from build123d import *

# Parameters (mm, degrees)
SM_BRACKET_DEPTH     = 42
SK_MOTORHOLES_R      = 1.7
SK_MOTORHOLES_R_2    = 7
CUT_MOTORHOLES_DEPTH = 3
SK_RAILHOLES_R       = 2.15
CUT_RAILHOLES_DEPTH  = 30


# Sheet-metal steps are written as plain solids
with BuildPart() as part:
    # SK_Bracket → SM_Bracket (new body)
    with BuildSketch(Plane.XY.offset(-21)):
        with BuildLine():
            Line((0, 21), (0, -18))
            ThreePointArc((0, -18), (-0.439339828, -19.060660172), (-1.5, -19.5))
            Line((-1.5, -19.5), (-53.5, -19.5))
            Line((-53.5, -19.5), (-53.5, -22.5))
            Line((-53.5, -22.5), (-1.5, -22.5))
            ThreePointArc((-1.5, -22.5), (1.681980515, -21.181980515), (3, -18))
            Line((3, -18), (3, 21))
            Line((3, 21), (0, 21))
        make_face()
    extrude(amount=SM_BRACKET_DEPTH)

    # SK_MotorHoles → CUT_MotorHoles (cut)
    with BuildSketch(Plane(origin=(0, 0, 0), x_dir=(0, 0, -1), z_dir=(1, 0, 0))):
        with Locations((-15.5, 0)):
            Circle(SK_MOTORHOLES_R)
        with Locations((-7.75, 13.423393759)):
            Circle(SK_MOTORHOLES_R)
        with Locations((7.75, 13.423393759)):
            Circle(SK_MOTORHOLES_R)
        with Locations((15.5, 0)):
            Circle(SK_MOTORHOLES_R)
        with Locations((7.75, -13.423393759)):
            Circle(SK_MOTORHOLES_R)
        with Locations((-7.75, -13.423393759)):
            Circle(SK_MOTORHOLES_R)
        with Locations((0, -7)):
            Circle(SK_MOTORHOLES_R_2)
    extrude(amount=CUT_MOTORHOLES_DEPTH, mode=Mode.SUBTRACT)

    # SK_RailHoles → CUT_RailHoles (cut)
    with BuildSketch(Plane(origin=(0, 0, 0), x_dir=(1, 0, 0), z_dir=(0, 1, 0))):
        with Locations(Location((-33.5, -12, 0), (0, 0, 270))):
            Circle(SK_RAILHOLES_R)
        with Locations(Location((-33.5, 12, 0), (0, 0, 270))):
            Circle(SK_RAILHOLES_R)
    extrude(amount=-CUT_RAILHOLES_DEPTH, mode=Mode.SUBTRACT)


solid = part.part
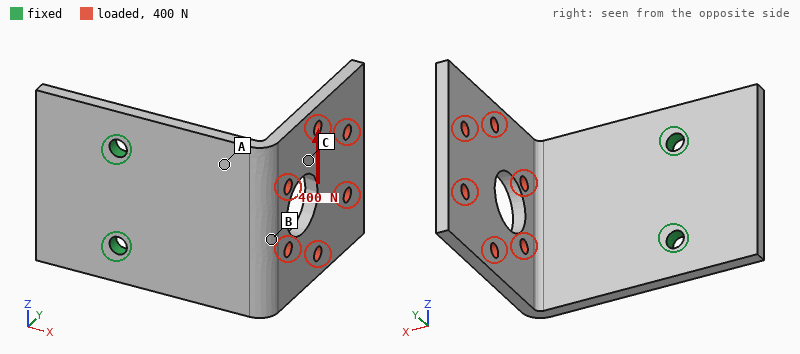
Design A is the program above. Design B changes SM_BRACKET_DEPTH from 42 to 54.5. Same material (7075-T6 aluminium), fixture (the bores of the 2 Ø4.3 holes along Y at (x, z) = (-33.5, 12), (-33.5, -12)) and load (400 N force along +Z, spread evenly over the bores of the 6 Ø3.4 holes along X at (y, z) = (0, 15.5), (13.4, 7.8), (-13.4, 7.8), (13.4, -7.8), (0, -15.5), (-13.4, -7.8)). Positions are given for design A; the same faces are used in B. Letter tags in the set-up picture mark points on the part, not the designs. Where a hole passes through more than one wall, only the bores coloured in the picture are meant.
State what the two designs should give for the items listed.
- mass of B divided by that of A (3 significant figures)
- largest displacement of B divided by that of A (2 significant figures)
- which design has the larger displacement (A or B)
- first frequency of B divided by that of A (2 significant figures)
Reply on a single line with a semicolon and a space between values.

1.32; 0.84; A; 0.97
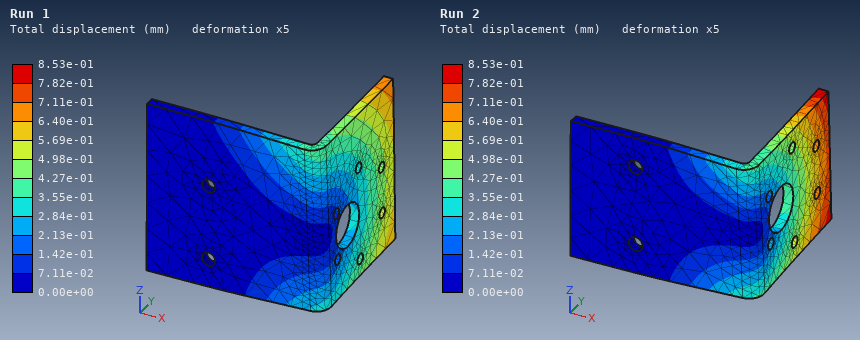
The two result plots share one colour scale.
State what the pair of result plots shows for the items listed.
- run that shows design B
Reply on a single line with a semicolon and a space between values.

Run 1
